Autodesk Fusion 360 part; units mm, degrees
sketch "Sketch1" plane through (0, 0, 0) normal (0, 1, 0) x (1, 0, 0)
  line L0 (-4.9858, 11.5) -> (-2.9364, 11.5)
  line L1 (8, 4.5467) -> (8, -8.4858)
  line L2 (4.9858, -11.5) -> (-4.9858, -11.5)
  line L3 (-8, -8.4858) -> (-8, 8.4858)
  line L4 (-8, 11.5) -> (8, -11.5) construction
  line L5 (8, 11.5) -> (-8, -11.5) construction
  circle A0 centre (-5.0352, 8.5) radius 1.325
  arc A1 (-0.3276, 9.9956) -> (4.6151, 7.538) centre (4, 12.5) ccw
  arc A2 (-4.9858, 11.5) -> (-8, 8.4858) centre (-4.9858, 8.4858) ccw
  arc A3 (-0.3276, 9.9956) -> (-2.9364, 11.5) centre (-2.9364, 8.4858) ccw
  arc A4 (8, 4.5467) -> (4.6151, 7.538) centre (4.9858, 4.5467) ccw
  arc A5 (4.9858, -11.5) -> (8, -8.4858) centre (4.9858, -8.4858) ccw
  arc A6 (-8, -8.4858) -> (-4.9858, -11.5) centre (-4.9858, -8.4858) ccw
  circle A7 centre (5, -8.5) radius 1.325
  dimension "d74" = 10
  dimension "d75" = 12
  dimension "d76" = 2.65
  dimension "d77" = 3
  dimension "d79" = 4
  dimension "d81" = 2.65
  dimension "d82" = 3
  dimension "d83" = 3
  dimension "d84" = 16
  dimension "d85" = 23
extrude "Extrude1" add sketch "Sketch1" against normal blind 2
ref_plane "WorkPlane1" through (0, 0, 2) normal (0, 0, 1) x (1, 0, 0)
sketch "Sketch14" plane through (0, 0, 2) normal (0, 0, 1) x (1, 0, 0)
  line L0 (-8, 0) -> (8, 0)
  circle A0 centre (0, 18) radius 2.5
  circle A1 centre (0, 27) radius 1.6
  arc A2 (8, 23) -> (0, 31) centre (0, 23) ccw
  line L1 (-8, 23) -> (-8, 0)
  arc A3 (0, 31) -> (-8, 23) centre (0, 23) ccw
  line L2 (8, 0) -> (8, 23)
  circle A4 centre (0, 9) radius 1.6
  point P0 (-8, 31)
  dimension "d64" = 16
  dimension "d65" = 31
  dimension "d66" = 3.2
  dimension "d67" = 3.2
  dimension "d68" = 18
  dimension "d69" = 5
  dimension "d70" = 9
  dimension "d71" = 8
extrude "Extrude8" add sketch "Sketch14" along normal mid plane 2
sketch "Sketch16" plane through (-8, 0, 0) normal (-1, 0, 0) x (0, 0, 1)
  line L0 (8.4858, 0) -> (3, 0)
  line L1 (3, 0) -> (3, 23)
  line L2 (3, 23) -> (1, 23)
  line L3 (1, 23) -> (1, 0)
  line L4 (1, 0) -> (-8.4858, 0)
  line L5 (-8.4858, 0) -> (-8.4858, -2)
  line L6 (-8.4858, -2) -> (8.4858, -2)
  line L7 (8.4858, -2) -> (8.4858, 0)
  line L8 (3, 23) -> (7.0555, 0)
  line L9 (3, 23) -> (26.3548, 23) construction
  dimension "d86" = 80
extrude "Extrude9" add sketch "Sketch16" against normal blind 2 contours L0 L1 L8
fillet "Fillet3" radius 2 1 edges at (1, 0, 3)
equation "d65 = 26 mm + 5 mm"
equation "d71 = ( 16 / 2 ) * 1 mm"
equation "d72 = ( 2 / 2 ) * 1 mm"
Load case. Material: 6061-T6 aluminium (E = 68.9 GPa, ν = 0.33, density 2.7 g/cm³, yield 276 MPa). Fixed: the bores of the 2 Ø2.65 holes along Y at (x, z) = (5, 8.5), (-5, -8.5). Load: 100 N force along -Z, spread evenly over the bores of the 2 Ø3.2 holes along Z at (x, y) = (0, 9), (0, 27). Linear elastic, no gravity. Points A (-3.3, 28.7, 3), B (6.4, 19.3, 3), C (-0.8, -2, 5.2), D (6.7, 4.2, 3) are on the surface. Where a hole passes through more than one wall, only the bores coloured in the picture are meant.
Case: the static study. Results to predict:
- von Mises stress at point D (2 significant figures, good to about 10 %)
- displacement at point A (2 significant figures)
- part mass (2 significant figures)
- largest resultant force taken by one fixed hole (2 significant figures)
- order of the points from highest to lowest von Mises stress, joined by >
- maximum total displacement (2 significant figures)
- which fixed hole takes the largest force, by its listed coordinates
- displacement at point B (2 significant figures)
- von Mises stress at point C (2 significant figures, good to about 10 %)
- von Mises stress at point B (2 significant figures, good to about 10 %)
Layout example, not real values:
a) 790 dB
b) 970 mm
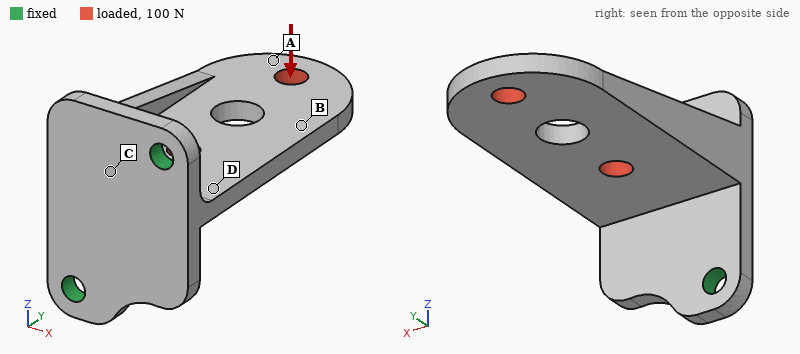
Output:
a) 79 MPa
b) 0.40 mm
c) 4.3 g
d) 130 N
e) D > C > B > A
f) 0.46 mm
g) (5, 8.5)
h) 0.25 mm
i) 57 MPa
j) 32 MPa
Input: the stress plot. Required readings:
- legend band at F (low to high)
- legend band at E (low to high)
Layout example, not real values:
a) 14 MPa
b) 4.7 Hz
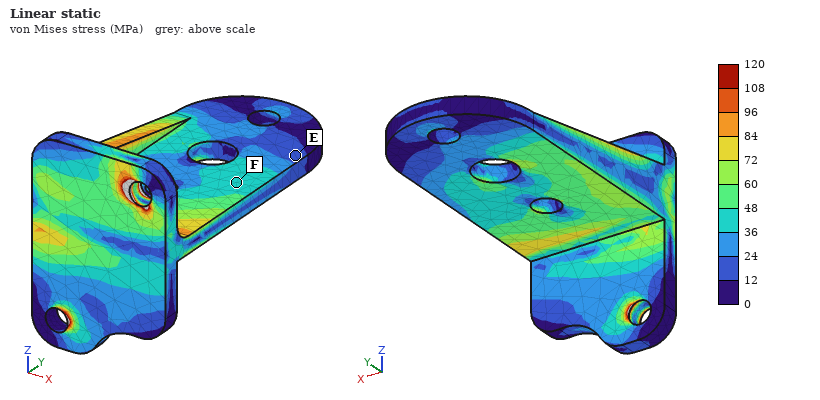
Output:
a) 36 to 48 MPa
b) 12 to 24 MPa
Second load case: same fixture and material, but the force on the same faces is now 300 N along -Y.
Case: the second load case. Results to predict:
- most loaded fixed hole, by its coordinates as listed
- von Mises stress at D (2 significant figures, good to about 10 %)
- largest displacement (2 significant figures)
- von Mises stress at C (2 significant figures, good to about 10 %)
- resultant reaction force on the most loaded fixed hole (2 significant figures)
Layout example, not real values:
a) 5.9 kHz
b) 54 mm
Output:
a) (5, 8.5)
b) 13 MPa
c) 48 µm
d) 23 MPa
e) 190 N
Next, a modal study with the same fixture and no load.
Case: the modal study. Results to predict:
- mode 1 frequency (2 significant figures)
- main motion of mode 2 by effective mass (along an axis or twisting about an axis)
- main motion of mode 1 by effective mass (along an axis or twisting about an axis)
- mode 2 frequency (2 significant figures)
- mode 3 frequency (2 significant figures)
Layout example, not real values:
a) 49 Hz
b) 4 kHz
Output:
a) 2200 Hz
b) along X
c) along Z
d) 3500 Hz
e) 7800 Hz
